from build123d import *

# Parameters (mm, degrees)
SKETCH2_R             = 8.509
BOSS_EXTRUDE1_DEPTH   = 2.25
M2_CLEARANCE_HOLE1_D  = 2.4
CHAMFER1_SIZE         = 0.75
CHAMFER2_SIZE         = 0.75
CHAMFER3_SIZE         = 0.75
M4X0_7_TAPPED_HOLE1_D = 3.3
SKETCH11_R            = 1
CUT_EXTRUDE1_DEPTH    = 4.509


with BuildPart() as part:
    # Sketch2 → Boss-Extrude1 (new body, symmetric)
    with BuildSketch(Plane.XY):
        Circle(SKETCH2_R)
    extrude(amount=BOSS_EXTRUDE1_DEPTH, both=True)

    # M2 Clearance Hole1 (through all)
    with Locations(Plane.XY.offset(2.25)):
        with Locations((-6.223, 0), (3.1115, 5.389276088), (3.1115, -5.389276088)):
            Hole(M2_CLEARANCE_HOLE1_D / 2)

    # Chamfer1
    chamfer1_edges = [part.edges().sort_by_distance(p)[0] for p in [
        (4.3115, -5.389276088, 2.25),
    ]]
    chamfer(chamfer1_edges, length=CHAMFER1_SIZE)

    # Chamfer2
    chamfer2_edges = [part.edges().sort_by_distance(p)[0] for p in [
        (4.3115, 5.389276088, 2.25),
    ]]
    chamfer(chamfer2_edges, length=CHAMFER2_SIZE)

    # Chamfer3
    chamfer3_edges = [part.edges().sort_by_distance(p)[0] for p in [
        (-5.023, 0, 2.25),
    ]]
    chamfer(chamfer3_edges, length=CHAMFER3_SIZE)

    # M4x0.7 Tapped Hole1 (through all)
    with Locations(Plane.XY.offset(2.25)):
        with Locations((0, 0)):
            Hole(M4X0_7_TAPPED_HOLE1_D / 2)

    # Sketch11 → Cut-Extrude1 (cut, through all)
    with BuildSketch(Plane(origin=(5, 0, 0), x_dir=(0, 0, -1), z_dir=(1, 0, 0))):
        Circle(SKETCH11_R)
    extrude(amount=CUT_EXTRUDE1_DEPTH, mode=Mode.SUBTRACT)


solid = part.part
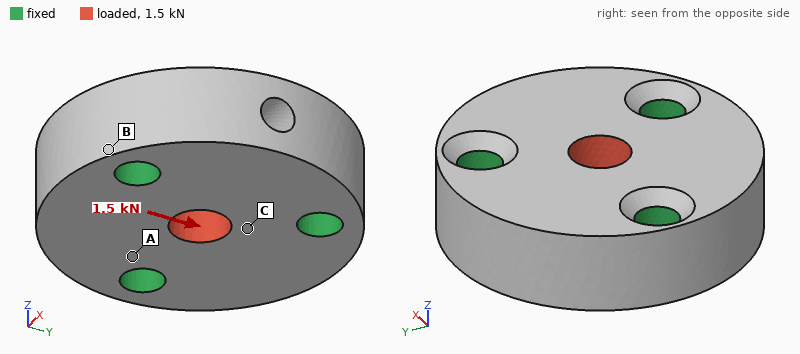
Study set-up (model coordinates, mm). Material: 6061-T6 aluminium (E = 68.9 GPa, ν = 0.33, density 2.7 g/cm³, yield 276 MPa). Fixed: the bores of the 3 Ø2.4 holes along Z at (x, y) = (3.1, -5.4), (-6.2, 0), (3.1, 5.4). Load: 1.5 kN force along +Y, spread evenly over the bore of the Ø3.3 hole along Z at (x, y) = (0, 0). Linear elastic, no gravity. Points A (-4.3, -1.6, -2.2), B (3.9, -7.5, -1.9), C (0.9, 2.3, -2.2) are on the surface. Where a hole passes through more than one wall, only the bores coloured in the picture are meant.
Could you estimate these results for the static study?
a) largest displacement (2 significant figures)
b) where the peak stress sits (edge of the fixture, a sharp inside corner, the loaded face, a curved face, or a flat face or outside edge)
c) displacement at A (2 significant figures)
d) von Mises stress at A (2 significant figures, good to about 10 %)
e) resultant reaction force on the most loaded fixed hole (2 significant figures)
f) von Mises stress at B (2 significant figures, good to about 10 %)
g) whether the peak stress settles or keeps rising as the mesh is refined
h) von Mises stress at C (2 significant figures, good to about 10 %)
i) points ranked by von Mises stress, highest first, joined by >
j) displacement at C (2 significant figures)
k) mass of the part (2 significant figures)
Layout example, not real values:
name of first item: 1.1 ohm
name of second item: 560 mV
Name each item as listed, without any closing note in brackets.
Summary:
largest displacement: 2.8 µm
where the peak stress sits: edge of the fixture
displacement at A: 0.81 µm
von Mises stress at A: 17 MPa
resultant reaction force on the most loaded fixed hole: 520 N
von Mises stress at B: 6.3 MPa
whether the peak stress settles or keeps rising as the mesh is refined: keeps rising
von Mises stress at C: 33 MPa
points ranked by von Mises stress, highest first, joined by >: C > A > B
displacement at C: 1.6 µm
mass of the part: 2.4 g
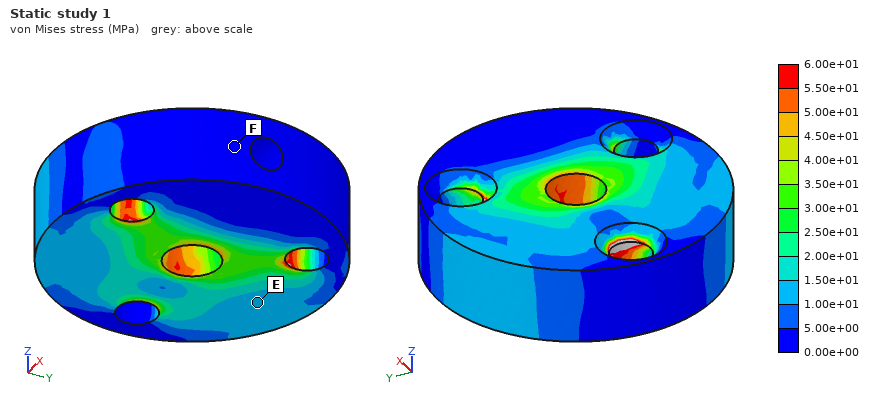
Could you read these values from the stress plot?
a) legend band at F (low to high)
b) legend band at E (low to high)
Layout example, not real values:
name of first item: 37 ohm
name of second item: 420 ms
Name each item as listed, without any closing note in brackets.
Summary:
legend band at F: 0.00e+00 to 5.00e+00 MPa
legend band at E: 1.00e+01 to 1.50e+01 MPa
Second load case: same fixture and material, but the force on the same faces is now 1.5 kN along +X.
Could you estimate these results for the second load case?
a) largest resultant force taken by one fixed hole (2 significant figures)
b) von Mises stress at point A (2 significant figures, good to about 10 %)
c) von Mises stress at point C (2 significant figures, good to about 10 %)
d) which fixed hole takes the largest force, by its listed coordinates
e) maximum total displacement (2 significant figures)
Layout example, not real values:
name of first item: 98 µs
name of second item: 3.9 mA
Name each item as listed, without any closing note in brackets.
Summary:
largest resultant force taken by one fixed hole: 550 N
von Mises stress at point A: 20 MPa
von Mises stress at point C: 21 MPa
which fixed hole takes the largest force, by its listed coordinates: (-6.2, 0)
maximum total displacement: 3.1 µm
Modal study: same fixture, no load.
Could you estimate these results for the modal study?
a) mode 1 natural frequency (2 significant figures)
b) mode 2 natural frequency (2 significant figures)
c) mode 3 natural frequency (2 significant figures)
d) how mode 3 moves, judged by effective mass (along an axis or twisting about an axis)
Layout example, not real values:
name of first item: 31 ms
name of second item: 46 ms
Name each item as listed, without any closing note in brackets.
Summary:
mode 1 natural frequency: 81 kHz
mode 2 natural frequency: 83 kHz
mode 3 natural frequency: 91 kHz
how mode 3 moves, judged by effective mass: along Z
